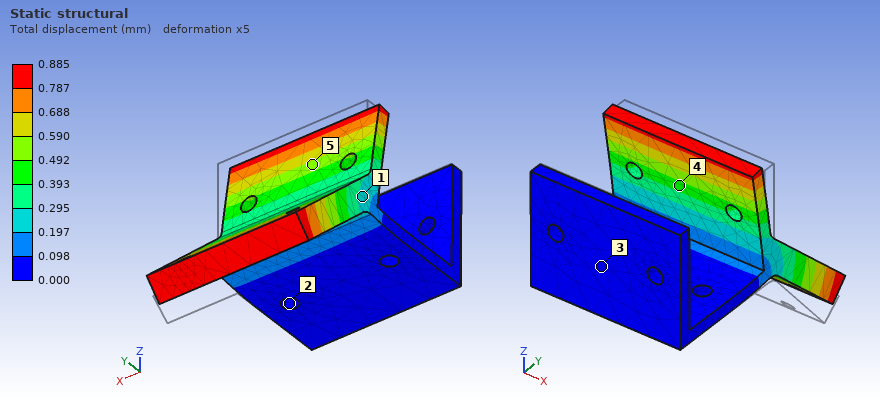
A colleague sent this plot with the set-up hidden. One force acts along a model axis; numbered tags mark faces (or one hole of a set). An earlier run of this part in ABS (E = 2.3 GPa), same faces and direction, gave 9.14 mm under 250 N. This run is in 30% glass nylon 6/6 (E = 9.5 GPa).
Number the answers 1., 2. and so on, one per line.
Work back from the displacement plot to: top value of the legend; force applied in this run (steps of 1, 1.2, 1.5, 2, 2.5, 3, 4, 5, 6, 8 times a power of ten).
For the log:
1. 0.885 mm
2. 100 N
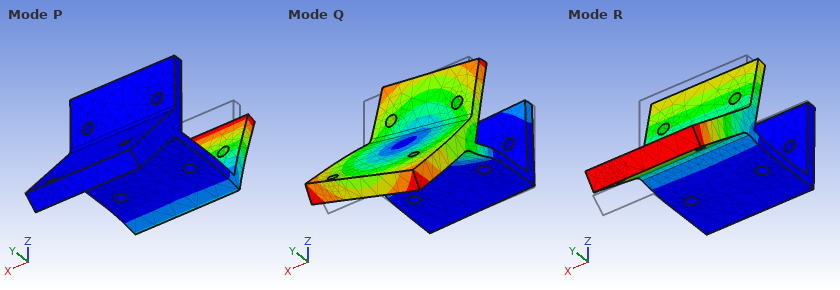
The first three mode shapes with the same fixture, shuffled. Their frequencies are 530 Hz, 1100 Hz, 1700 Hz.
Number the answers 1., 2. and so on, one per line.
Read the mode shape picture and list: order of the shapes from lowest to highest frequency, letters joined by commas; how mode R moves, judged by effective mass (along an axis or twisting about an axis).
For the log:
1. R, P, Q
2. along Z
